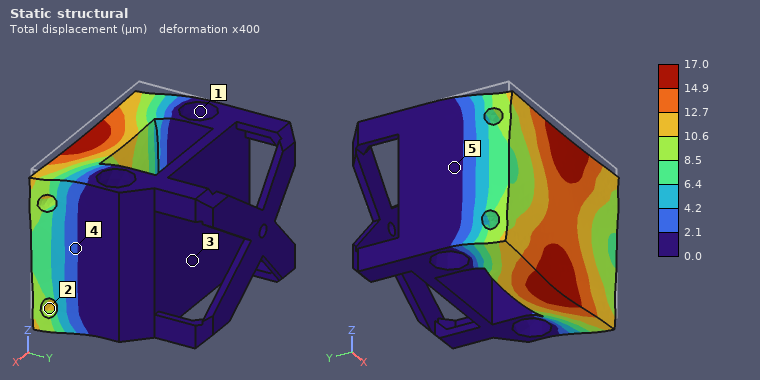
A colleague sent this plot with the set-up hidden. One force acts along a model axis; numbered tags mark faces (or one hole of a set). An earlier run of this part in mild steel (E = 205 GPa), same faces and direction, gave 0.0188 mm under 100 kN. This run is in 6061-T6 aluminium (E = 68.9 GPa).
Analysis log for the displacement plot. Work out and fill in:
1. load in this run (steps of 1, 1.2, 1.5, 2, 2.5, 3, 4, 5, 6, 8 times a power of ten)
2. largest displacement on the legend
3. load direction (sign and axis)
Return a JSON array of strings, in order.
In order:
["30 kN", "17.0 µm", "-Z"]
